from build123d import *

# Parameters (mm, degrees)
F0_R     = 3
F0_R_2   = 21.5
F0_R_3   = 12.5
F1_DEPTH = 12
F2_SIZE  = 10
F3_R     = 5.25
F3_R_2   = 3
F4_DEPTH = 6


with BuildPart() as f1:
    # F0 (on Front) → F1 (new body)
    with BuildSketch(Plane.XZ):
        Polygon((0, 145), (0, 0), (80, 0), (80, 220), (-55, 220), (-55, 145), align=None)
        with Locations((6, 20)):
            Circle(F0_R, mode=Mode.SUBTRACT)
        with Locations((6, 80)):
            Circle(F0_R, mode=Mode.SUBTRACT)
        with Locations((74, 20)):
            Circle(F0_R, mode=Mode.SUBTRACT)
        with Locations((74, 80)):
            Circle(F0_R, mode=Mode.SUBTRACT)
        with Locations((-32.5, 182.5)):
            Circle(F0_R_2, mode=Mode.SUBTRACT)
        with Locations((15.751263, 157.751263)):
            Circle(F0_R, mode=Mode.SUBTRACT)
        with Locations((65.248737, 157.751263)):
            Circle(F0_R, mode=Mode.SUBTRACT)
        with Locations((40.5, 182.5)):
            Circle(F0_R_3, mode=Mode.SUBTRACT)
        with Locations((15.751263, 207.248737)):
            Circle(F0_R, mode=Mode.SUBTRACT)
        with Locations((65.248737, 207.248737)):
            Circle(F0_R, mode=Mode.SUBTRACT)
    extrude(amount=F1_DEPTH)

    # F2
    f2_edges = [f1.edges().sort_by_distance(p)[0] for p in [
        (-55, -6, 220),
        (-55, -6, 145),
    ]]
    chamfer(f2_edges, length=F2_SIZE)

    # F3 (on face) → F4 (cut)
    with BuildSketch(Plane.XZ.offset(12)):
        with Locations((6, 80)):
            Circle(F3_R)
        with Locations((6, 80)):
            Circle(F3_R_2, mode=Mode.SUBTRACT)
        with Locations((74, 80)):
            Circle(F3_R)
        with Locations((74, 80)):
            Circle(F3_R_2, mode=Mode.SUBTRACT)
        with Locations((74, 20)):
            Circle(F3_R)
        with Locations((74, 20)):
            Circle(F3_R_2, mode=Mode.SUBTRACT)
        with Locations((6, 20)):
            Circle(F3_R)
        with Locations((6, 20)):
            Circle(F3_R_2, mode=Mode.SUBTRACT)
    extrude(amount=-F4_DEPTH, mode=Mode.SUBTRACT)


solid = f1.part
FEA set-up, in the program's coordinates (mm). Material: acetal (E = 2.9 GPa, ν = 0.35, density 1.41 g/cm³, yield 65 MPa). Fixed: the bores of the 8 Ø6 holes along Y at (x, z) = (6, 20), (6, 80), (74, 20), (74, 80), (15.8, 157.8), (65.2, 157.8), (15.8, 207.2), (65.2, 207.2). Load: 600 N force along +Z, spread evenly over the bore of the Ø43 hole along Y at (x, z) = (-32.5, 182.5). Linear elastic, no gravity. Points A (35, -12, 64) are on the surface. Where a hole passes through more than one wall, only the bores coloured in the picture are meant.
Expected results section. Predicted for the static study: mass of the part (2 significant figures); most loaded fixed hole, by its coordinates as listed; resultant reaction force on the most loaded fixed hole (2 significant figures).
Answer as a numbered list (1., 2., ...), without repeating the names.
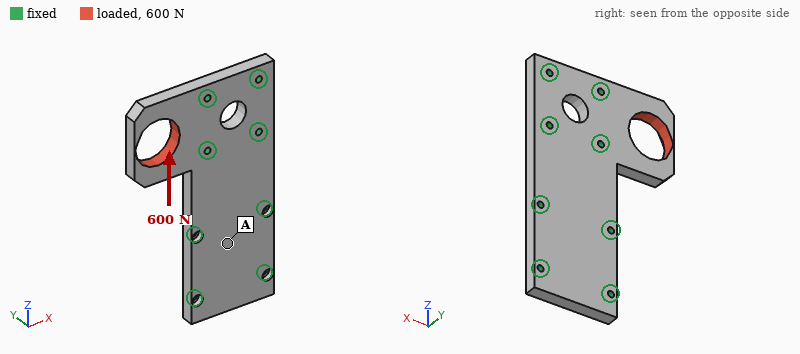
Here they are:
1. 330 g
2. (15.8, 207.2)
3. 480 N
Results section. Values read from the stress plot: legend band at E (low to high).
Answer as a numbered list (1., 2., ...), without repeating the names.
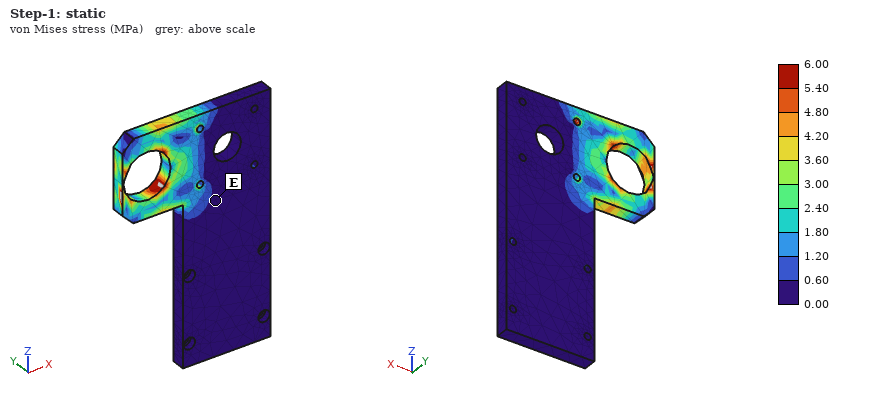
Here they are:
1. 0.00 to 0.60 MPa
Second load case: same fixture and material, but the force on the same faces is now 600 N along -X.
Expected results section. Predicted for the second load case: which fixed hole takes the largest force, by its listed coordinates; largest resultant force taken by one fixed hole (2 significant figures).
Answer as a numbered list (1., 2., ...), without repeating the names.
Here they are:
1. (15.8, 207.2)
2. 280 N
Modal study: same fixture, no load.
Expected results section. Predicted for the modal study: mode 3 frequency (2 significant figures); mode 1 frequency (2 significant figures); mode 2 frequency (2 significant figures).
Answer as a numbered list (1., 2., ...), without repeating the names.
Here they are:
1. 1600 Hz
2. 650 Hz
3. 1100 Hz
